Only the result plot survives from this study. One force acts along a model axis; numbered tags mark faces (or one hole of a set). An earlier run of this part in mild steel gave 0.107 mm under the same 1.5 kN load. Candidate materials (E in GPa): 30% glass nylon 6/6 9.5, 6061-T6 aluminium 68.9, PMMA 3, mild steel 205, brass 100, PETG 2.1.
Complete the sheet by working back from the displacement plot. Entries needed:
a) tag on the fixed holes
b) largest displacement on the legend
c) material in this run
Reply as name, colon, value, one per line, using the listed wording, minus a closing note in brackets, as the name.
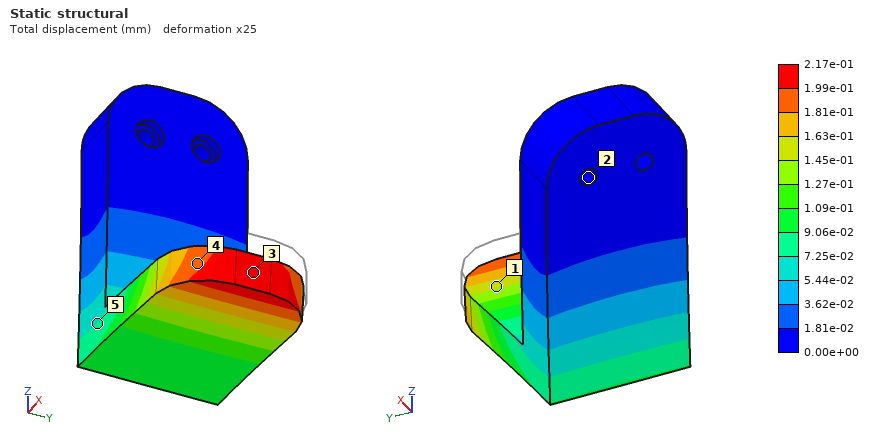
tag on the fixed holes: 2
largest displacement on the legend: 2.17e-01 mm
material in this run: brass
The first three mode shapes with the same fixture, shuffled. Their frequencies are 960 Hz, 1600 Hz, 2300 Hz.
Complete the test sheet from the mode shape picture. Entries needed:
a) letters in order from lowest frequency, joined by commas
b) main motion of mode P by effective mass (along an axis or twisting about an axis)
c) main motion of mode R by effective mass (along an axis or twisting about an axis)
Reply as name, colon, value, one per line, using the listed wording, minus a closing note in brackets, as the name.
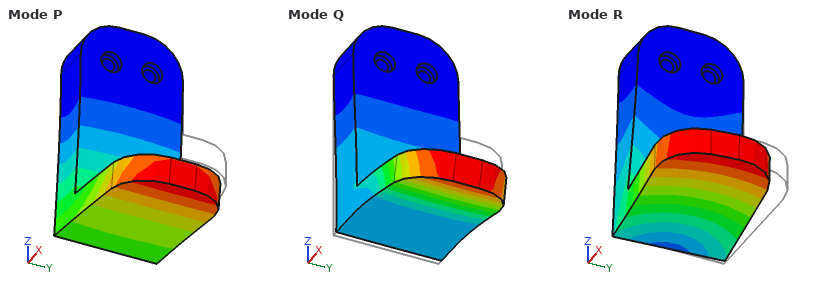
letters in order from lowest frequency, joined by commas: P, R, Q
main motion of mode P by effective mass: along X
main motion of mode R by effective mass: along Y
